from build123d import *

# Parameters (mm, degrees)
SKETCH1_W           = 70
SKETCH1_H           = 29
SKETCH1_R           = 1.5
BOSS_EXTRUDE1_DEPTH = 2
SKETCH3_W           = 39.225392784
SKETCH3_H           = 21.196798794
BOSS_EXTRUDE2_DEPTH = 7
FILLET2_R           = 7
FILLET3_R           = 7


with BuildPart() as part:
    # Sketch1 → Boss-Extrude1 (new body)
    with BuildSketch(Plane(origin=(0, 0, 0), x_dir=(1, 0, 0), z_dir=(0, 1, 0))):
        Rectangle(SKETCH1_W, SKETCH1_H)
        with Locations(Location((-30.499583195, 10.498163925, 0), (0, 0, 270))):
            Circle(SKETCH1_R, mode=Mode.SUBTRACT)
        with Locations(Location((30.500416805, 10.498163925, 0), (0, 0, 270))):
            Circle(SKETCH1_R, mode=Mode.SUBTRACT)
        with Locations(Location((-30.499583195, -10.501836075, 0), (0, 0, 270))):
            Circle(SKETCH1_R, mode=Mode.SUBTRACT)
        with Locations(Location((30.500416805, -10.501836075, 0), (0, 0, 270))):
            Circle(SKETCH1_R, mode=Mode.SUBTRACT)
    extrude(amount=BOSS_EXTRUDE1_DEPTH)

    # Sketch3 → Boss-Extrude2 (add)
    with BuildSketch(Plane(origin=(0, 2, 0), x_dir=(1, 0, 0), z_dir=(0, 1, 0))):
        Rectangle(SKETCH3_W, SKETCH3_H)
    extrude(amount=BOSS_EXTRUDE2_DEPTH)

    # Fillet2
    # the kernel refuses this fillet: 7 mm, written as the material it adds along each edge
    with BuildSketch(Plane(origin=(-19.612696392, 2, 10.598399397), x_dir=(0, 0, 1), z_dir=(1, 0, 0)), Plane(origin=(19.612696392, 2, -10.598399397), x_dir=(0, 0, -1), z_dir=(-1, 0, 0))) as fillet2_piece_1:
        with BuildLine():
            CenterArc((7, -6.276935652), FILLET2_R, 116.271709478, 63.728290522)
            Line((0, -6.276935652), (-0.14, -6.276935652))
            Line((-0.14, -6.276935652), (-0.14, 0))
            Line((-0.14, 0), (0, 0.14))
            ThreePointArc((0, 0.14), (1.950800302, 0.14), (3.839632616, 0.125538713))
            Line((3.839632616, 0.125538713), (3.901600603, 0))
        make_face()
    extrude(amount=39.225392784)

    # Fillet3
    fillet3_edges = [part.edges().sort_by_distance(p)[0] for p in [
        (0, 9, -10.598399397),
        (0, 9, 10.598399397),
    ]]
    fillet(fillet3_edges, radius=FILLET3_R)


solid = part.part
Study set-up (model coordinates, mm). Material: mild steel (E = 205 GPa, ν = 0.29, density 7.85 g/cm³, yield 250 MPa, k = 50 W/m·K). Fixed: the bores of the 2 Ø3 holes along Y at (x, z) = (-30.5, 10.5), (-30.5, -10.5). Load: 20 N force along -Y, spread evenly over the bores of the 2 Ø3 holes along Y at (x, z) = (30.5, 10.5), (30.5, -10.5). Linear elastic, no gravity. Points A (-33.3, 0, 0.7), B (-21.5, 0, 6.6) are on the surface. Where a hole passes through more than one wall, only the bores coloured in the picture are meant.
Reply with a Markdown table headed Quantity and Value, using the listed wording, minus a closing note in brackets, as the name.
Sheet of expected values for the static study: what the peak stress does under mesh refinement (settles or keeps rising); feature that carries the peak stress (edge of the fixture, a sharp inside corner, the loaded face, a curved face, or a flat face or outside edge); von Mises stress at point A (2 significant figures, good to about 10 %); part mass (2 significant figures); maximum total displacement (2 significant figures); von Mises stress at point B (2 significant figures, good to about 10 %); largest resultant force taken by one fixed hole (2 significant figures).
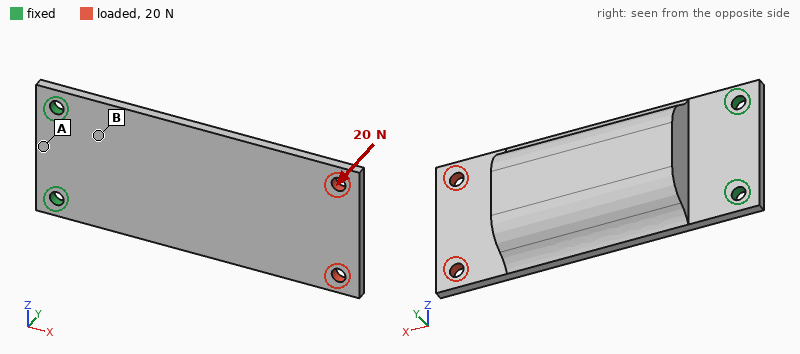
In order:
| Quantity | Value |
|---|---|
| what the peak stress does under mesh refinement | keeps rising |
| feature that carries the peak stress | edge of the fixture |
| von Mises stress at point A | 13 MPa |
| part mass | 78 g |
| maximum total displacement | 0.20 mm |
| von Mises stress at point B | 48 MPa |
| largest resultant force taken by one fixed hole | 11 N |
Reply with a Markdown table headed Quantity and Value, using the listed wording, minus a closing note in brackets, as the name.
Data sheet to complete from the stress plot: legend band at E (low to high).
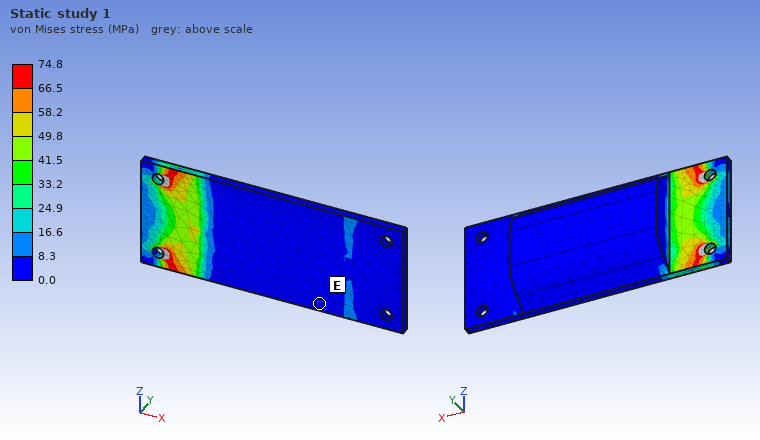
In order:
| Quantity | Value |
|---|---|
| legend band at E | 0.0 to 8.3 MPa |
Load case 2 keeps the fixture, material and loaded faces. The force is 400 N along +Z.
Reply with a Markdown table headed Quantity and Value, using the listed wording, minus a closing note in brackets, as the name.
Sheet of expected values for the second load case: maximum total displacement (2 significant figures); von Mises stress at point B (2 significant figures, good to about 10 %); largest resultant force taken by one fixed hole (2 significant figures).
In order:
| Quantity | Value |
|---|---|
| maximum total displacement | 38 µm |
| von Mises stress at point B | 37 MPa |
| largest resultant force taken by one fixed hole | 1.1 kN |
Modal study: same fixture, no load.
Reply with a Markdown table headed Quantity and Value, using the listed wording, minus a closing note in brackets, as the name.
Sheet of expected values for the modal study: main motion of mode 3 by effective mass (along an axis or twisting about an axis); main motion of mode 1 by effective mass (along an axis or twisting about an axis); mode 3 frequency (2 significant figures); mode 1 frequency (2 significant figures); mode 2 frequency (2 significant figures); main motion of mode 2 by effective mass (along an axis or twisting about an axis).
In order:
| Quantity | Value |
|---|---|
| main motion of mode 3 by effective mass | along Z |
| main motion of mode 1 by effective mass | along Y |
| mode 3 frequency | 4000 Hz |
| mode 1 frequency | 360 Hz |
| mode 2 frequency | 3400 Hz |
| main motion of mode 2 by effective mass | along Z |
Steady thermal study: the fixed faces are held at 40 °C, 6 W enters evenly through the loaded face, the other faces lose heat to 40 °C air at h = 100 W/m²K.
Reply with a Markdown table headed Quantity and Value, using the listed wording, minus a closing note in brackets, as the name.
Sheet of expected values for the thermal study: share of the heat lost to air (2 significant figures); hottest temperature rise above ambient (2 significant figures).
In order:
| Quantity | Value |
|---|---|
| share of the heat lost to air | 84 % |
| hottest temperature rise above ambient | 38 K |
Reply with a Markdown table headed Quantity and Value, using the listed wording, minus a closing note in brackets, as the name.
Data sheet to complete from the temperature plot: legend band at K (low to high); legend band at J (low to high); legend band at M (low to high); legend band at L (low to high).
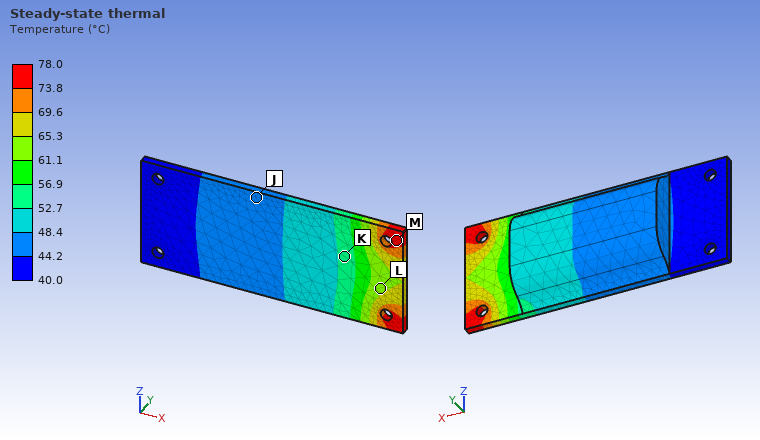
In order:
| Quantity | Value |
|---|---|
| legend band at K | 52.7 to 56.9 °C |
| legend band at J | 44.2 to 48.4 °C |
| legend band at M | 73.8 to 78.0 °C |
| legend band at L | 61.1 to 65.3 °C |
